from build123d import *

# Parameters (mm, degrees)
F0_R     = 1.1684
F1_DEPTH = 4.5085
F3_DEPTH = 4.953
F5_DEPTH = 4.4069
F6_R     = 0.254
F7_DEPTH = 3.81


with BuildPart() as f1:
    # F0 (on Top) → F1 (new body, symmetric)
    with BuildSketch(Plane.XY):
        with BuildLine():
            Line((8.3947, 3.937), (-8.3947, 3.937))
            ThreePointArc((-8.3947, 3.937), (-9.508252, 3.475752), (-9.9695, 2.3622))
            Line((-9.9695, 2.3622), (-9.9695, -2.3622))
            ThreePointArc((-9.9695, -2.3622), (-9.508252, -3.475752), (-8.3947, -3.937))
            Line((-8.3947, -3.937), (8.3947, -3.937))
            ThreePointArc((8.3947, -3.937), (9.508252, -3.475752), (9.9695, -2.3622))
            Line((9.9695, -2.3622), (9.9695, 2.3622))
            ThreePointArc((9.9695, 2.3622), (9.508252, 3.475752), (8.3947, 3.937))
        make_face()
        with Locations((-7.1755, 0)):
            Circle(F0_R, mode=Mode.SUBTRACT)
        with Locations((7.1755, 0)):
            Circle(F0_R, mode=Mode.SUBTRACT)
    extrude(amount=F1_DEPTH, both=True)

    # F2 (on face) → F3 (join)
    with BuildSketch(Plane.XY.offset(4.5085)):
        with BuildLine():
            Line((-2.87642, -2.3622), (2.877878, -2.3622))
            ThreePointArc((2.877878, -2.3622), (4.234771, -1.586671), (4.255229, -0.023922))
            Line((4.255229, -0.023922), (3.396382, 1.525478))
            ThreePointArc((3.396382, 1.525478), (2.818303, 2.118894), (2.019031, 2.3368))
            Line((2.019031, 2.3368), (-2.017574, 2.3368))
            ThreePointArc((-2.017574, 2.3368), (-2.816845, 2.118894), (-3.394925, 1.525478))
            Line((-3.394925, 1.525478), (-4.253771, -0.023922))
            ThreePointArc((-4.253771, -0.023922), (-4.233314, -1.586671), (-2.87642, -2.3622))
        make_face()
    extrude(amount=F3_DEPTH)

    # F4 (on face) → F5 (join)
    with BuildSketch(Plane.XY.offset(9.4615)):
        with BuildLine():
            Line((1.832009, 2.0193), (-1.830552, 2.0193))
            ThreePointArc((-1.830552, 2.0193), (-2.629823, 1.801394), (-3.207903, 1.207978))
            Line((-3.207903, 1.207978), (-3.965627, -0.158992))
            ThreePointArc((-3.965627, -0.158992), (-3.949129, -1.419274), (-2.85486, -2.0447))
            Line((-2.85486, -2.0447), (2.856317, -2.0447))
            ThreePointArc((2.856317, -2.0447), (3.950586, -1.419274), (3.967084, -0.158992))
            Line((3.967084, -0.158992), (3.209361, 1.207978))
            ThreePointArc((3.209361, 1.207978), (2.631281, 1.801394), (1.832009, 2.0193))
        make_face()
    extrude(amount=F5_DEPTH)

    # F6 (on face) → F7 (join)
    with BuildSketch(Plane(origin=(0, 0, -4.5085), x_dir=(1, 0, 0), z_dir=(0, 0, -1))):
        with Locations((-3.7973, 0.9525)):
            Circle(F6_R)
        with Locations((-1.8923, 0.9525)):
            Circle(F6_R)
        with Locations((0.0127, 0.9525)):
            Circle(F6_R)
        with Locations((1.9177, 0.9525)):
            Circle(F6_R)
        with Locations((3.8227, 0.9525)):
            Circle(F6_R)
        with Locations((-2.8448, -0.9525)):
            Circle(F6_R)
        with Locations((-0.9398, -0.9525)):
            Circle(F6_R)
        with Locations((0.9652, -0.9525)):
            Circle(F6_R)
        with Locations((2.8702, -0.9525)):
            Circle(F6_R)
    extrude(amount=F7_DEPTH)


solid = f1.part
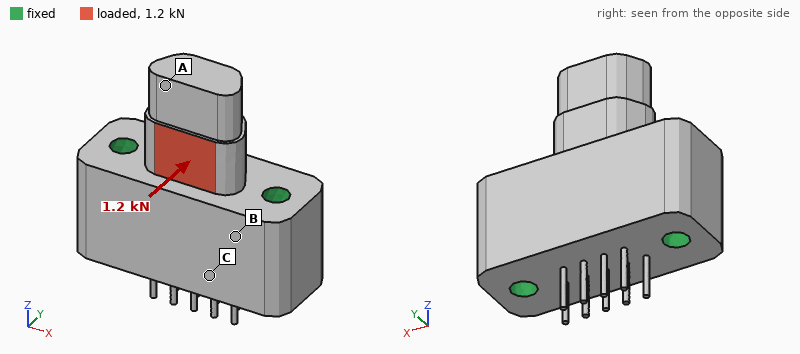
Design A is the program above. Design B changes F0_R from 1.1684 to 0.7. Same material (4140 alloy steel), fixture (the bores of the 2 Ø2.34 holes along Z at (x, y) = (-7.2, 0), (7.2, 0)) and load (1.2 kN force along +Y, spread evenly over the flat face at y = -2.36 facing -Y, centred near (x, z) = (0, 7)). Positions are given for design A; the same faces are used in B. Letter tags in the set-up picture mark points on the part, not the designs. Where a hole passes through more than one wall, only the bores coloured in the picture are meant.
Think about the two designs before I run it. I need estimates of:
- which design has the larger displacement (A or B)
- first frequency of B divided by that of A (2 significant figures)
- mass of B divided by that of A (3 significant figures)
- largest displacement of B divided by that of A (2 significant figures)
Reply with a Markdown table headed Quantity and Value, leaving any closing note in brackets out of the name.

| Quantity | Value |
|---|---|
| which design has the larger displacement | B |
| first frequency of B divided by that of A | 1.0 |
| mass of B divided by that of A | 1.03 |
| largest displacement of B divided by that of A | 1.1 |
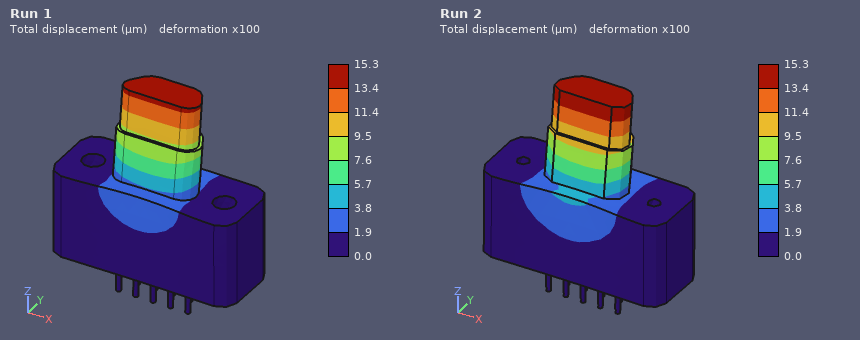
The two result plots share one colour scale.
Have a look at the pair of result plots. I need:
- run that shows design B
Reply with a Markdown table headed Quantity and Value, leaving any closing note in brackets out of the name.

| Quantity | Value |
|---|---|
| run that shows design B | Run 2 |
